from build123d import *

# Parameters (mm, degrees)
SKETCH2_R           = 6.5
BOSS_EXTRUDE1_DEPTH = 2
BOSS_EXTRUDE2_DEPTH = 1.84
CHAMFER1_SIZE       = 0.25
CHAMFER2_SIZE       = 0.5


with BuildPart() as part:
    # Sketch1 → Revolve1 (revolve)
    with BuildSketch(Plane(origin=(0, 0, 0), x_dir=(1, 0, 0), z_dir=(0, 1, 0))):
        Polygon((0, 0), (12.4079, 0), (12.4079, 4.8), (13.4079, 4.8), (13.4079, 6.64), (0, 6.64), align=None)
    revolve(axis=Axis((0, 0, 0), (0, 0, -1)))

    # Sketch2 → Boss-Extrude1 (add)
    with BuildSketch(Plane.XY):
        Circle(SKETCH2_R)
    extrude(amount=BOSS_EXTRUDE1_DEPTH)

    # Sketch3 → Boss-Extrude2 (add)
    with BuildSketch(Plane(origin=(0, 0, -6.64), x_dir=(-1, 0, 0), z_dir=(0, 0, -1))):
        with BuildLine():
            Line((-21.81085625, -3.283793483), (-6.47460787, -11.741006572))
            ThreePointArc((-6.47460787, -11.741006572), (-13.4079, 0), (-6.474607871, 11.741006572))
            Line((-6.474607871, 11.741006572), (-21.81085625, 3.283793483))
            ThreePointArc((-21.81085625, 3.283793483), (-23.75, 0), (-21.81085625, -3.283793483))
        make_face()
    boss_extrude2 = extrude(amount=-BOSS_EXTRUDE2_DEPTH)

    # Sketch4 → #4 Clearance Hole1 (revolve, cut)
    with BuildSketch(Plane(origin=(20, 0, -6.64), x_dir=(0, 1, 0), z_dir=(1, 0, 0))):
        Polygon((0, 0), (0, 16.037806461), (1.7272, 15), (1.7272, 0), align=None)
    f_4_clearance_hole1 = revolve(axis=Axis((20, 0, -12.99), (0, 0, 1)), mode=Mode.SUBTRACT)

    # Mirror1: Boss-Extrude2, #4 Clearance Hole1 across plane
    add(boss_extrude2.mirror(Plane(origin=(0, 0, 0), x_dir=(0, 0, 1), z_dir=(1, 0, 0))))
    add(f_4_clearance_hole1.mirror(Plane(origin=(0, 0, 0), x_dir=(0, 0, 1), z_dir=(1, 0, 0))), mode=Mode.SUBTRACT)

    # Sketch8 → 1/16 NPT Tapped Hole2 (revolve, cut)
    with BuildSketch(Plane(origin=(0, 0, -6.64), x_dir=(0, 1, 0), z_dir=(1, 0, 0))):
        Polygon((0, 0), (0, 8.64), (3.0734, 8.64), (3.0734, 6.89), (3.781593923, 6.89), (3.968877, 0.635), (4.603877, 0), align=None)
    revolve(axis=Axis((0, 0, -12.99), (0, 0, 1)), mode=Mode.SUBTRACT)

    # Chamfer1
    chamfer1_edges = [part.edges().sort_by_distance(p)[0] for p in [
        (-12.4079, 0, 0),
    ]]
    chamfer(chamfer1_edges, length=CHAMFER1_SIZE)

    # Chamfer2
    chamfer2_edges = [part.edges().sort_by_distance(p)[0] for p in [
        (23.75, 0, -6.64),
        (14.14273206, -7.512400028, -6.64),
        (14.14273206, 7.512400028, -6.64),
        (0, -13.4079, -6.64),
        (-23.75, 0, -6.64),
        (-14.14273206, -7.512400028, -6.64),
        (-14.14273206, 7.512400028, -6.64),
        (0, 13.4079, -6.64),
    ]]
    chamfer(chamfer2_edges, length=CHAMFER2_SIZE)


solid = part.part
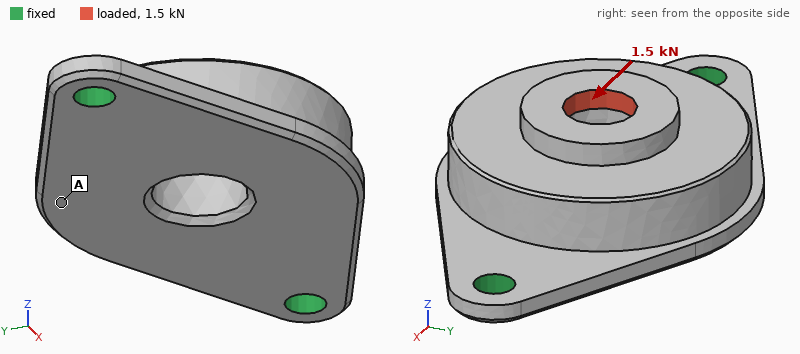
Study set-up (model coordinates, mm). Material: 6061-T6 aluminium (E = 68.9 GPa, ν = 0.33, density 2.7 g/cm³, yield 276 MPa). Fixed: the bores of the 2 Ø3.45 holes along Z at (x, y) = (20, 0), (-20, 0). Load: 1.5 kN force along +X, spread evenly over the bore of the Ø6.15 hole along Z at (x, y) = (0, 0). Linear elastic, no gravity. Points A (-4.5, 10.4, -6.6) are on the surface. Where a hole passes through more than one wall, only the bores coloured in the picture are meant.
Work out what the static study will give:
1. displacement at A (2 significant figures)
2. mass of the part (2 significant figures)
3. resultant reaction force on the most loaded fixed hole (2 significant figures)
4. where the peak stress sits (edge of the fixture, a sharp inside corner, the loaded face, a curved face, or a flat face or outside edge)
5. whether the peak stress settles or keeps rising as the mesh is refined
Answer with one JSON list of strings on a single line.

["11 µm", "9.8 g", "820 N", "edge of the fixture", "keeps rising"]
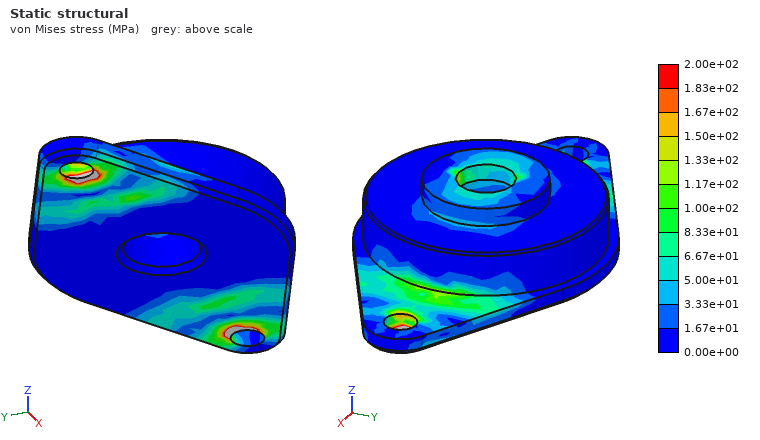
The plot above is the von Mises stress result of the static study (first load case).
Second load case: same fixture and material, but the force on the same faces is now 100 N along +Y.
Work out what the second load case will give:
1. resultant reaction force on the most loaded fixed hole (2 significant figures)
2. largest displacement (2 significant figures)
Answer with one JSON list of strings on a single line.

["50 N", "42 µm"]
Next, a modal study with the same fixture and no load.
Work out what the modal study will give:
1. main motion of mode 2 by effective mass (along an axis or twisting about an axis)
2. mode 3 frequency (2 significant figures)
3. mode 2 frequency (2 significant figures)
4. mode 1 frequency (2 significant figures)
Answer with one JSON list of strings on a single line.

["along Z", "14 kHz", "6500 Hz", "3500 Hz"]
